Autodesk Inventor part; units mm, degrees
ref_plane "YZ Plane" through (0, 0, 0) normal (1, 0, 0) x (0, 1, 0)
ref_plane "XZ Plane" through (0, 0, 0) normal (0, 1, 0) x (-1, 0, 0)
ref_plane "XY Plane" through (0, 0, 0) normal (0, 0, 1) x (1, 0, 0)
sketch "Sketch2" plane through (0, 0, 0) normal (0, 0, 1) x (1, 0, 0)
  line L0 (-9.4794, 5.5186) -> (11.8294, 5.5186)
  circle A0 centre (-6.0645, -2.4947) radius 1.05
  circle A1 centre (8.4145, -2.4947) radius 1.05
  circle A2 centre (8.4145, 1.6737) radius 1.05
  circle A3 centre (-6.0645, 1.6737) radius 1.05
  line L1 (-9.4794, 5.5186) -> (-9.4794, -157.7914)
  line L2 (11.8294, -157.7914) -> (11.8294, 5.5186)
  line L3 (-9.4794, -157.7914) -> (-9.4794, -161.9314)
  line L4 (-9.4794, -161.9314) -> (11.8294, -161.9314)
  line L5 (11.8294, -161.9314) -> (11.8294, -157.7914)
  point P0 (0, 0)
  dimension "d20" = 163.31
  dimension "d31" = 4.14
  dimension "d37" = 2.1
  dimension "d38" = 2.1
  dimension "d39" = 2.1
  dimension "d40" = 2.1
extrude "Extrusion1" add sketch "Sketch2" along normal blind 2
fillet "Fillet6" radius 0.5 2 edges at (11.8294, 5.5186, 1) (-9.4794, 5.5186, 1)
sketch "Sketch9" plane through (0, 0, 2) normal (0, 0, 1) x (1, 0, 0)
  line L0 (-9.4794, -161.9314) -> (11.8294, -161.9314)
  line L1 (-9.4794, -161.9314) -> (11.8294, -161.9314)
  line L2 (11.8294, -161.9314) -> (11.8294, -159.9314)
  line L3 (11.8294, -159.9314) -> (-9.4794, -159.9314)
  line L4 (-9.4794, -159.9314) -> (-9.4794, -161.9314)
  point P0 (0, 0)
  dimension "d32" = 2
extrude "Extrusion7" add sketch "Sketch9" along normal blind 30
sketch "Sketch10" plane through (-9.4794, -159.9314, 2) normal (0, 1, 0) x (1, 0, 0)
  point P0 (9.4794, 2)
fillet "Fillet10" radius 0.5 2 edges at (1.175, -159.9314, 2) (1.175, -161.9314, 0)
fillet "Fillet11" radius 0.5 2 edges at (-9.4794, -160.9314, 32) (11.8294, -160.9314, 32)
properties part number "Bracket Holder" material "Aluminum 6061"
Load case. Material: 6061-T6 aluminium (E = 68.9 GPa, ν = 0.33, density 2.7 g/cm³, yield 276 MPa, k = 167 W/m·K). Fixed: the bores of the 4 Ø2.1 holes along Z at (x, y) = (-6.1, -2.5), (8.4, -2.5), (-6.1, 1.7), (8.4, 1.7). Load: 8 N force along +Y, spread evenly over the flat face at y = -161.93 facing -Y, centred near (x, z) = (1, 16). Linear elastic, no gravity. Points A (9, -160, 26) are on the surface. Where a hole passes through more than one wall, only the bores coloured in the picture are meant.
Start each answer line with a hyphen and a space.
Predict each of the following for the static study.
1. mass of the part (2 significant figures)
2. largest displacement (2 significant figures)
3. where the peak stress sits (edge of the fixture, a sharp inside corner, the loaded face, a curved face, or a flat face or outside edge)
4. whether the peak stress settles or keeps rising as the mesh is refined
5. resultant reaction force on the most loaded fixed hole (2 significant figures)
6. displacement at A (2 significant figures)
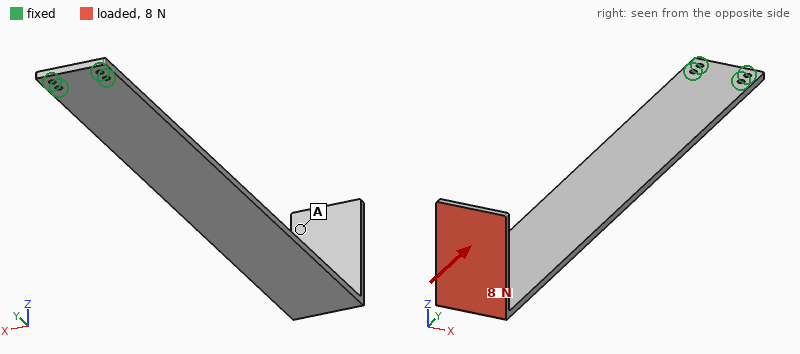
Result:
- 23 g
- 1.7 mm
- edge of the fixture
- keeps rising
- 5.5 N
- 1.6 mm
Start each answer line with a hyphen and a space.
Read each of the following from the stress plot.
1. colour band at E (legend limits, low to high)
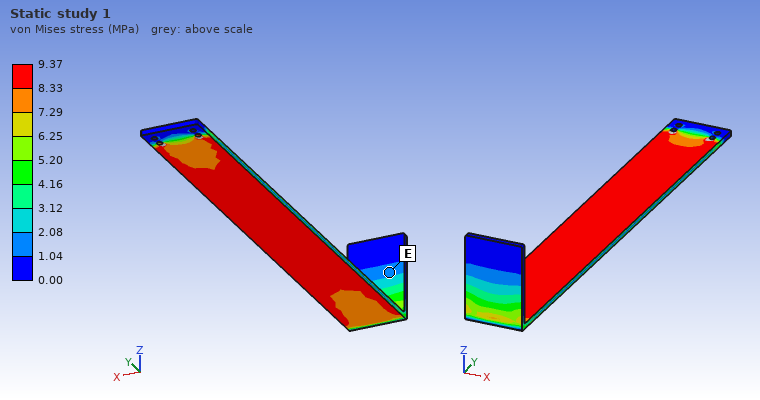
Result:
- 1.04 to 2.08 MPa
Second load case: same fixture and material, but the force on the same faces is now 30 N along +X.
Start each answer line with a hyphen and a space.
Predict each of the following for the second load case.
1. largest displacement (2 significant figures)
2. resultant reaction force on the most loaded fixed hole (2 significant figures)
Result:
- 1.9 mm
- 260 N
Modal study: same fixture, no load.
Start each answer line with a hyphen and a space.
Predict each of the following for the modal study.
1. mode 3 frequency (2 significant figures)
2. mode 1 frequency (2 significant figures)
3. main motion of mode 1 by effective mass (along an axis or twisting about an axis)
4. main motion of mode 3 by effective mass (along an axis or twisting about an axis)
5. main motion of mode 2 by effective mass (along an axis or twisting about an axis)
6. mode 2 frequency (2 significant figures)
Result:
- 360 Hz
- 48 Hz
- along Z
- along X
- along Z
- 310 Hz
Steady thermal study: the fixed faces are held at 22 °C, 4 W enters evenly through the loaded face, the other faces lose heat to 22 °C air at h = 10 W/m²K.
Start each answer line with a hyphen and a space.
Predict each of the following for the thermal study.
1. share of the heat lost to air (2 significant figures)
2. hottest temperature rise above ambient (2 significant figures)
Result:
- 55 %
- 60 K
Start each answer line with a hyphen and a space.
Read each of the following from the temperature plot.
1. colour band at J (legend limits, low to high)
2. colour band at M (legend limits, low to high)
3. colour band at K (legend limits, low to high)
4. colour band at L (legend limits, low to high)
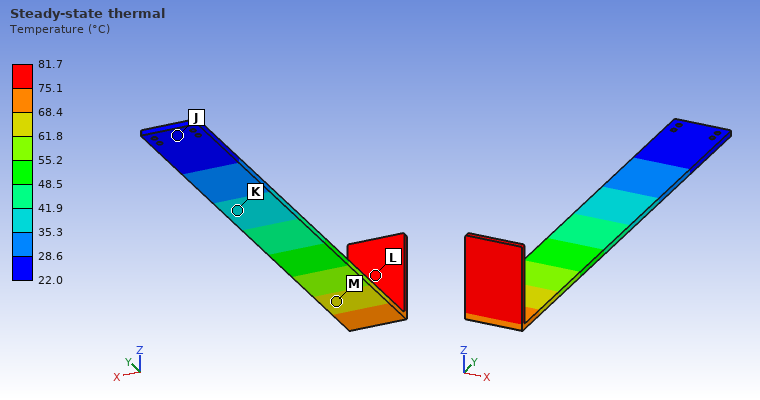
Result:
- 22.0 to 28.6 °C
- 61.8 to 68.4 °C
- 35.3 to 41.9 °C
- 75.1 to 81.7 °C
